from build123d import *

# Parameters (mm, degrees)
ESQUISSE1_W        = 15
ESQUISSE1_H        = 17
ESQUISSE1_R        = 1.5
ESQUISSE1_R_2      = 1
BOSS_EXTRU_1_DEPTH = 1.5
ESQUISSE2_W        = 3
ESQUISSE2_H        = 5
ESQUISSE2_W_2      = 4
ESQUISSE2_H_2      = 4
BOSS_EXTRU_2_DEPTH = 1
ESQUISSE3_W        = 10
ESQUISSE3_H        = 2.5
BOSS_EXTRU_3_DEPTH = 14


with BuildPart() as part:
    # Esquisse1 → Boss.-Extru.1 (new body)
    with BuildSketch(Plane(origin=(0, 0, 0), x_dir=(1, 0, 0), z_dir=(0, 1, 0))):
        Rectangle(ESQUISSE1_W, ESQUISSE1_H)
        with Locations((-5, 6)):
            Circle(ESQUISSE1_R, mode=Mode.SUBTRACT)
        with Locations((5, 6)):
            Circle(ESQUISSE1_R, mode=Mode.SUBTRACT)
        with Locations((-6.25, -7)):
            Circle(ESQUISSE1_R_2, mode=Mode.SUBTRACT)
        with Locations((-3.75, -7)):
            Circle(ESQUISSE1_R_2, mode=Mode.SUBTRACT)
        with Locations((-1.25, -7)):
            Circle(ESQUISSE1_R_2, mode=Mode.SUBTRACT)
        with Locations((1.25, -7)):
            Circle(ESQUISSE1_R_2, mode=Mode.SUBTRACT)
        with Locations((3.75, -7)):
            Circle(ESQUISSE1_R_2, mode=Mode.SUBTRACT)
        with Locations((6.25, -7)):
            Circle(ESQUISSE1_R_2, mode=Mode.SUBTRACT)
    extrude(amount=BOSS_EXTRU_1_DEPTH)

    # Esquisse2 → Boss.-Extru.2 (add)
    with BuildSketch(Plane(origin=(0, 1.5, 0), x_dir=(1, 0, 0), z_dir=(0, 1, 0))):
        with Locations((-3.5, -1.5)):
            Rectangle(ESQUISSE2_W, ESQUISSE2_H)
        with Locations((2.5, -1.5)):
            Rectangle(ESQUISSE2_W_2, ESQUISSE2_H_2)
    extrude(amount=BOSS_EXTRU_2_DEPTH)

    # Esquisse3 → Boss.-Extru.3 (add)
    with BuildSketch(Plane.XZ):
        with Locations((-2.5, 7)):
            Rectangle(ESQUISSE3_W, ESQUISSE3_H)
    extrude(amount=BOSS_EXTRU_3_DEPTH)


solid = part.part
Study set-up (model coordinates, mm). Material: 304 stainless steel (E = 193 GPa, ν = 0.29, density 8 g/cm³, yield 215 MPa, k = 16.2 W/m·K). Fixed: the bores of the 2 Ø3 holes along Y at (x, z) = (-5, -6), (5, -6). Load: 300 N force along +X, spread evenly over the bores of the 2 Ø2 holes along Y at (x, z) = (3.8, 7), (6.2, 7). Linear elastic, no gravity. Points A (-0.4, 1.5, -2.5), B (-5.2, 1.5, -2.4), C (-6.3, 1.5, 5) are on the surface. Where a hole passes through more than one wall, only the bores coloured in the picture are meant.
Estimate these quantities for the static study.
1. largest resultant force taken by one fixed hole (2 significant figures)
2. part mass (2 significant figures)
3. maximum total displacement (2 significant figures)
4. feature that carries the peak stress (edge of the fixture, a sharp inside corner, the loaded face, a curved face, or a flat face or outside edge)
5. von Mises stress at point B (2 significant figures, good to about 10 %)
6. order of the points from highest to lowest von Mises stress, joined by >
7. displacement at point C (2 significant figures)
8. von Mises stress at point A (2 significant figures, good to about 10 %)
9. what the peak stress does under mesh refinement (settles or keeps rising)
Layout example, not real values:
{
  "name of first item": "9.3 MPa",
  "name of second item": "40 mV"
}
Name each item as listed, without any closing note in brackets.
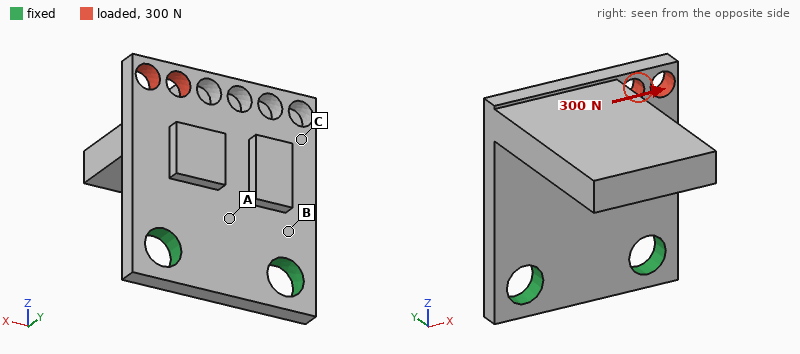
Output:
{
  "largest resultant force taken by one fixed hole": "370 N",
  "part mass": "5.7 g",
  "maximum total displacement": "8.8 µm",
  "feature that carries the peak stress": "a sharp inside corner",
  "von Mises stress at point B": "45 MPa",
  "order of the points from highest to lowest von Mises stress, joined by >": "B > A > C",
  "displacement at point C": "3.7 µm",
  "von Mises stress at point A": "28 MPa",
  "what the peak stress does under mesh refinement": "keeps rising"
}
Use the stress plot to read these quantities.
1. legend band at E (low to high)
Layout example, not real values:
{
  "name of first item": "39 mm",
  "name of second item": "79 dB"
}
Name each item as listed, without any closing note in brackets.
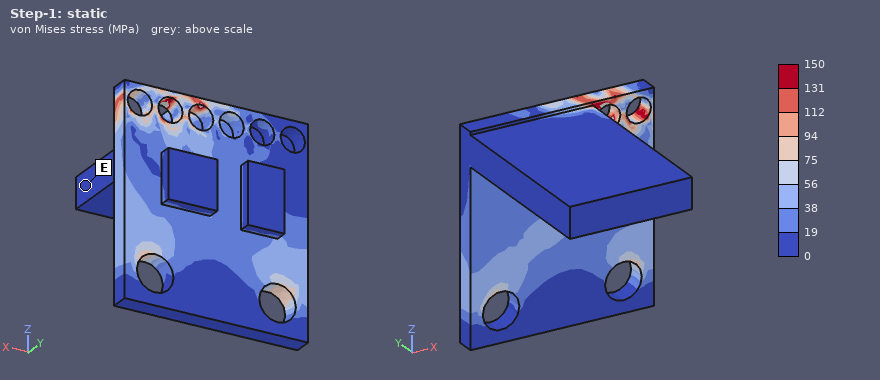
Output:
{
  "legend band at E": "0 to 19 MPa"
}
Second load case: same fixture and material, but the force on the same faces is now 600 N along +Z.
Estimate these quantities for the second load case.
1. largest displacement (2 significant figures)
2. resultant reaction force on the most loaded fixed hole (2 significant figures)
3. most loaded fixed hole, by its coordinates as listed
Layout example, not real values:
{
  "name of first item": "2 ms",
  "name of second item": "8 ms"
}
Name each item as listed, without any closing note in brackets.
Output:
{
  "largest displacement": "8.9 µm",
  "resultant reaction force on the most loaded fixed hole": "580 N",
  "most loaded fixed hole, by its coordinates as listed": "(5, -6)"
}
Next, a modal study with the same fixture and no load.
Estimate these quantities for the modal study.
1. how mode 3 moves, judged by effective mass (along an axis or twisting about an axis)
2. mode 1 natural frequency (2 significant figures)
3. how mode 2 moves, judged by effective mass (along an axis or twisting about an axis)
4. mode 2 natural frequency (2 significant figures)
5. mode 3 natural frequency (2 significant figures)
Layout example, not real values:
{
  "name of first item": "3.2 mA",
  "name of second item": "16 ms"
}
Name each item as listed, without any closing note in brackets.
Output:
{
  "how mode 3 moves, judged by effective mass": "along Y",
  "mode 1 natural frequency": "2200 Hz",
  "how mode 2 moves, judged by effective mass": "along X",
  "mode 2 natural frequency": "4300 Hz",
  "mode 3 natural frequency": "6400 Hz"
}
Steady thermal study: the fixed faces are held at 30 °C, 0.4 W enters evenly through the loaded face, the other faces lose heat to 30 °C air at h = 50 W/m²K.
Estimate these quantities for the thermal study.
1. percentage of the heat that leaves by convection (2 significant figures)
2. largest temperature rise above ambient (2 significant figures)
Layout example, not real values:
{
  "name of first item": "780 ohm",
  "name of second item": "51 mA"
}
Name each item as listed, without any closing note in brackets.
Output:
{
  "percentage of the heat that leaves by convection": "46 %",
  "largest temperature rise above ambient": "21 K"
}
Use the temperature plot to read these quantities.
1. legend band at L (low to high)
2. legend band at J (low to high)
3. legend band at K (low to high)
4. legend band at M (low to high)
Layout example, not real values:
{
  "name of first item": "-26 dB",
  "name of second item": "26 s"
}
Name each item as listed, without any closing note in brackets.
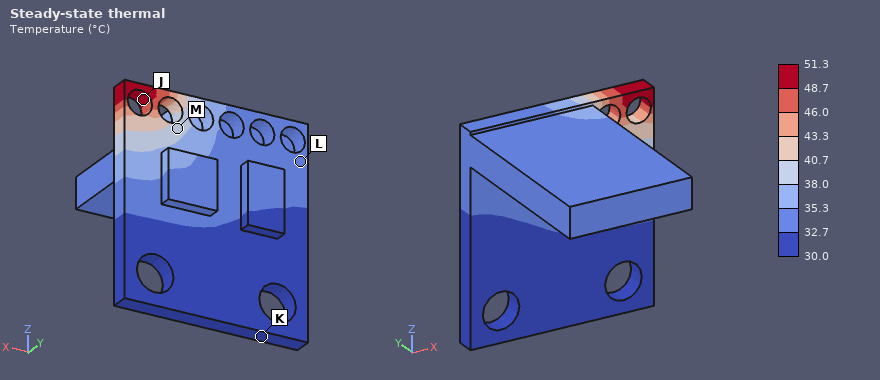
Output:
{
  "legend band at L": "32.7 to 35.3 °C",
  "legend band at J": "48.7 to 51.3 °C",
  "legend band at K": "30.0 to 32.7 °C",
  "legend band at M": "38.0 to 40.7 °C"
}
